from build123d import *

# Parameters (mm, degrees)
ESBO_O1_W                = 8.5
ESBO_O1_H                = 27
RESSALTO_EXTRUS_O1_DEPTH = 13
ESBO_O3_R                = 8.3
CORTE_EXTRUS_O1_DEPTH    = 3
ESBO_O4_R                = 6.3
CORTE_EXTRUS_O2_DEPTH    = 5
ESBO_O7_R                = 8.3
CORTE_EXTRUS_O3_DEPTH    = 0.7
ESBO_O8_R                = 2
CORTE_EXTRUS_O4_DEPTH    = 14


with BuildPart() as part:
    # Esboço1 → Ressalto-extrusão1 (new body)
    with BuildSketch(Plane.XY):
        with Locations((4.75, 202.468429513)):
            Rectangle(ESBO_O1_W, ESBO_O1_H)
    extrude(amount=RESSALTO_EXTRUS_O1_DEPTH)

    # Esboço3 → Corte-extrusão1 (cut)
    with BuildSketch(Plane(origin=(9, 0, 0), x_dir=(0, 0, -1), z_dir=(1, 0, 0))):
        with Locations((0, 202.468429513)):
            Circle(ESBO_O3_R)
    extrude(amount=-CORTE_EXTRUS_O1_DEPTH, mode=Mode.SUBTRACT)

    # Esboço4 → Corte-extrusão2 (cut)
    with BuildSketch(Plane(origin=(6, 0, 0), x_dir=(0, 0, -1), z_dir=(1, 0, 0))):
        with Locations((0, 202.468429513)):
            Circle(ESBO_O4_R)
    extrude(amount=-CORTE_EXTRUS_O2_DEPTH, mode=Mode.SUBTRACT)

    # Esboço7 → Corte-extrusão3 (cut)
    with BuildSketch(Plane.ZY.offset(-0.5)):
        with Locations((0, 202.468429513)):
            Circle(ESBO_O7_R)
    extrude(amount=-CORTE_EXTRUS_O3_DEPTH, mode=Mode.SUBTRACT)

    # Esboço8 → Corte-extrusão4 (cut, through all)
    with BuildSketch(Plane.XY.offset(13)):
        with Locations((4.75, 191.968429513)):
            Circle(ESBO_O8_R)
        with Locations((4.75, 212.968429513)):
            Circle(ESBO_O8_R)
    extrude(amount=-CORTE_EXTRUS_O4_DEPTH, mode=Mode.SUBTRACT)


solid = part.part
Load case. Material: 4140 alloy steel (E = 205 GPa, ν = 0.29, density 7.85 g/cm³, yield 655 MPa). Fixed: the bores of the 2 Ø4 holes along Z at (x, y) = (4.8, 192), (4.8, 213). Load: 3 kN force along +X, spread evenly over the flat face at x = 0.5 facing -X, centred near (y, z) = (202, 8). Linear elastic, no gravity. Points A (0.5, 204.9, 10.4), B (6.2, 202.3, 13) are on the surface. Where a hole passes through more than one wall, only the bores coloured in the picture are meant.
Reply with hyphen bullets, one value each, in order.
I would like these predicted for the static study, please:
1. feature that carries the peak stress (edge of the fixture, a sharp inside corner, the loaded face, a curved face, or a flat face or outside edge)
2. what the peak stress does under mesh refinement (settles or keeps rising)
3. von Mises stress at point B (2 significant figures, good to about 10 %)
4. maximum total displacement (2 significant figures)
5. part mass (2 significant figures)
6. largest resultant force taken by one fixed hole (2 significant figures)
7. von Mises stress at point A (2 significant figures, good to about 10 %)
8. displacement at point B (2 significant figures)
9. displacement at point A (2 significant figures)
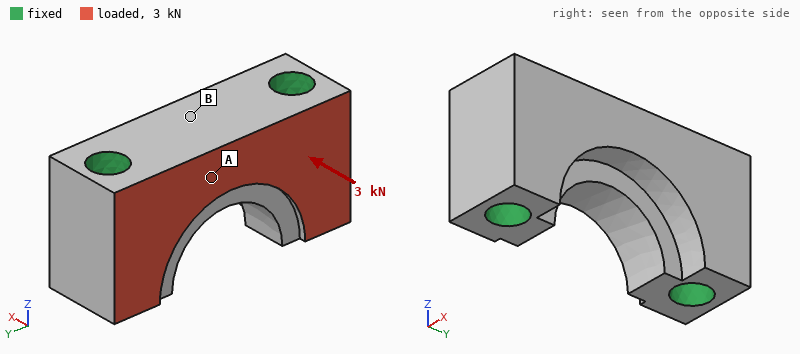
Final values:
- edge of the fixture
- keeps rising
- 5.5 MPa
- 1.6 µm
- 15 g
- 1.5 kN
- 15 MPa
- 1.4 µm
- 1.3 µm
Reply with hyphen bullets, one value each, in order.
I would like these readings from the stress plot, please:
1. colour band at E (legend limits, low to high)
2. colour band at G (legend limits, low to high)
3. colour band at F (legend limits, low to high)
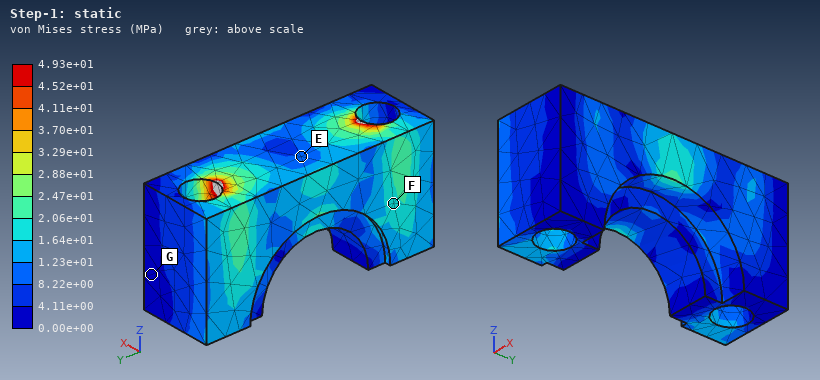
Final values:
- 8.22e+00 to 1.23e+01 MPa
- 0.00e+00 to 4.11e+00 MPa
- 1.64e+01 to 2.06e+01 MPa
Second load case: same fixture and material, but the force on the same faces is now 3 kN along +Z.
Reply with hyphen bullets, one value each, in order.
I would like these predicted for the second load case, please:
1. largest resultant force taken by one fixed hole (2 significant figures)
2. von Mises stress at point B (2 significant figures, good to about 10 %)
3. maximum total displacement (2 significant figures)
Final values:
- 1.5 kN
- 10 MPa
- 2.5 µm
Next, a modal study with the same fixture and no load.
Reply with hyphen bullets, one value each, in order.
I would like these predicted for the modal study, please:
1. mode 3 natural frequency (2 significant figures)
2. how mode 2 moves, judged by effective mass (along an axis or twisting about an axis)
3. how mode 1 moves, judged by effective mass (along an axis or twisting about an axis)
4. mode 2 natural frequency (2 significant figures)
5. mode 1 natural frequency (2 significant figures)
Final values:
- 100 kHz
- along Z
- along X
- 82 kHz
- 66 kHz
